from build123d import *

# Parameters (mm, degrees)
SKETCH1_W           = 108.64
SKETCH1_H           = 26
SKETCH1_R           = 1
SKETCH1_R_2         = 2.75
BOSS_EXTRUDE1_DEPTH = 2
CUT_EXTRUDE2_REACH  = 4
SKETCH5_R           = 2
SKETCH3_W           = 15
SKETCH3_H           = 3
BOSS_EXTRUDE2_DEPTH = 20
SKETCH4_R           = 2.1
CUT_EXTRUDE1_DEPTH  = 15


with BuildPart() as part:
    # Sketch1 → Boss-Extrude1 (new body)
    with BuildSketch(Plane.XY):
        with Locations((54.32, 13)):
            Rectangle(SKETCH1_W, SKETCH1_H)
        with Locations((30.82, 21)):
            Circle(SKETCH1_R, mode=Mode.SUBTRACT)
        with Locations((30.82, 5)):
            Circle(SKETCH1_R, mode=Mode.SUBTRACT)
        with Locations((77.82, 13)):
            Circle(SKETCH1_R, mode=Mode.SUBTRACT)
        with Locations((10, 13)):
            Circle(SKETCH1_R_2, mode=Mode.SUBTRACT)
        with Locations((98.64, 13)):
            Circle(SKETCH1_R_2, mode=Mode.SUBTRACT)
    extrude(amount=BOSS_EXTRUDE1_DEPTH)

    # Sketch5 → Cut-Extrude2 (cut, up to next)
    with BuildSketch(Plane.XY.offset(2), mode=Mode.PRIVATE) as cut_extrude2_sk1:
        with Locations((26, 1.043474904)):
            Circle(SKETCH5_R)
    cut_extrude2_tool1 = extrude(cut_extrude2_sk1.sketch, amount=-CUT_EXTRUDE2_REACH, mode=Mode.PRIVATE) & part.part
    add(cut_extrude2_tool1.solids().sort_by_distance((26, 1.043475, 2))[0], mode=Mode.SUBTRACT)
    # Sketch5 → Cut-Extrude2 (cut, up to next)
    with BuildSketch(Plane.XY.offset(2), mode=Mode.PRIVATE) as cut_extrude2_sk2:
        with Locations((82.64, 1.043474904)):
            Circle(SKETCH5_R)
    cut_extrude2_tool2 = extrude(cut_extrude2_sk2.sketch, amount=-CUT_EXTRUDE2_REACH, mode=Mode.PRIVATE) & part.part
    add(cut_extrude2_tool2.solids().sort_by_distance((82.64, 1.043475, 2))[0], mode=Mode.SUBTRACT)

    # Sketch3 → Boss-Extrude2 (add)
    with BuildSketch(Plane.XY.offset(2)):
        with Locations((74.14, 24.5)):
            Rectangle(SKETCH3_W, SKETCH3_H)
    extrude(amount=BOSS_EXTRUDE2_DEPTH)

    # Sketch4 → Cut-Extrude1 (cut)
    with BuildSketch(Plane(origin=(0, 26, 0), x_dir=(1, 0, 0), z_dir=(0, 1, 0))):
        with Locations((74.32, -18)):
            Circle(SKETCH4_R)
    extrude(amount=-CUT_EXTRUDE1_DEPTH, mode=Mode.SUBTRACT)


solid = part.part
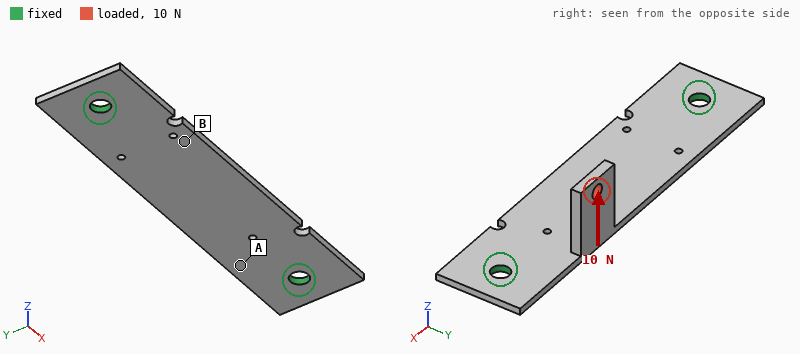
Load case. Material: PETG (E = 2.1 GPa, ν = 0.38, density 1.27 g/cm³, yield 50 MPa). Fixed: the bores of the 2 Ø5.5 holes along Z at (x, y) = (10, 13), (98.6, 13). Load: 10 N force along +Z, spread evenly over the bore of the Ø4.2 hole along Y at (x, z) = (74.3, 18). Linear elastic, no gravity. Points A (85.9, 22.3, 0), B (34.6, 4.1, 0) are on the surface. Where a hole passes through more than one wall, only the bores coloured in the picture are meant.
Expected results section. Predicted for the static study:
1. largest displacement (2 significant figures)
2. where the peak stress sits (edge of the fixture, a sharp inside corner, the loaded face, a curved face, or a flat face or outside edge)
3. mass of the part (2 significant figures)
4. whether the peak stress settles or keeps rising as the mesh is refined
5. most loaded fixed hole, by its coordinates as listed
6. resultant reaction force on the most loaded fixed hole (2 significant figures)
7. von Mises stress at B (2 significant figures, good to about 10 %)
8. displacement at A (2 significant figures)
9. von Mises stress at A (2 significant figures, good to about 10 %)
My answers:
1.1 mm
edge of the fixture
8.1 g
keeps rising
(98.6, 13)
8.1 N
1.1 MPa
0.32 mm
3.7 MPa
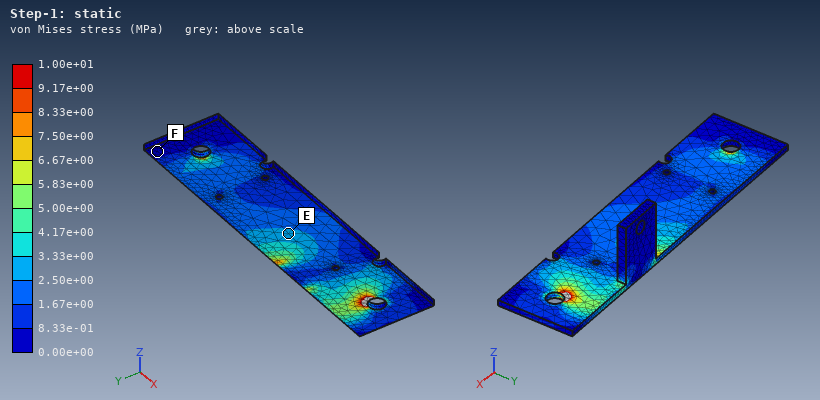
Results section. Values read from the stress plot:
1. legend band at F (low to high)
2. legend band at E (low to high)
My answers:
0.00e+00 to 8.33e-01 MPa
2.50e+00 to 3.33e+00 MPa
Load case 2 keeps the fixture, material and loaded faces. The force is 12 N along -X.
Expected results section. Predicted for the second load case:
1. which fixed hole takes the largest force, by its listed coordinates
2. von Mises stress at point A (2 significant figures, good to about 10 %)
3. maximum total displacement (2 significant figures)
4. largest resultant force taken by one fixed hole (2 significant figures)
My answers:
(98.6, 13)
5.0 MPa
1.1 mm
8.8 N
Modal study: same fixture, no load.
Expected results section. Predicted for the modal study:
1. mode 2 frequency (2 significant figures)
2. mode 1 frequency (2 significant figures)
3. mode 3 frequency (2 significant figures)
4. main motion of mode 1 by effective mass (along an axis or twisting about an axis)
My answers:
460 Hz
310 Hz
920 Hz
along Z
